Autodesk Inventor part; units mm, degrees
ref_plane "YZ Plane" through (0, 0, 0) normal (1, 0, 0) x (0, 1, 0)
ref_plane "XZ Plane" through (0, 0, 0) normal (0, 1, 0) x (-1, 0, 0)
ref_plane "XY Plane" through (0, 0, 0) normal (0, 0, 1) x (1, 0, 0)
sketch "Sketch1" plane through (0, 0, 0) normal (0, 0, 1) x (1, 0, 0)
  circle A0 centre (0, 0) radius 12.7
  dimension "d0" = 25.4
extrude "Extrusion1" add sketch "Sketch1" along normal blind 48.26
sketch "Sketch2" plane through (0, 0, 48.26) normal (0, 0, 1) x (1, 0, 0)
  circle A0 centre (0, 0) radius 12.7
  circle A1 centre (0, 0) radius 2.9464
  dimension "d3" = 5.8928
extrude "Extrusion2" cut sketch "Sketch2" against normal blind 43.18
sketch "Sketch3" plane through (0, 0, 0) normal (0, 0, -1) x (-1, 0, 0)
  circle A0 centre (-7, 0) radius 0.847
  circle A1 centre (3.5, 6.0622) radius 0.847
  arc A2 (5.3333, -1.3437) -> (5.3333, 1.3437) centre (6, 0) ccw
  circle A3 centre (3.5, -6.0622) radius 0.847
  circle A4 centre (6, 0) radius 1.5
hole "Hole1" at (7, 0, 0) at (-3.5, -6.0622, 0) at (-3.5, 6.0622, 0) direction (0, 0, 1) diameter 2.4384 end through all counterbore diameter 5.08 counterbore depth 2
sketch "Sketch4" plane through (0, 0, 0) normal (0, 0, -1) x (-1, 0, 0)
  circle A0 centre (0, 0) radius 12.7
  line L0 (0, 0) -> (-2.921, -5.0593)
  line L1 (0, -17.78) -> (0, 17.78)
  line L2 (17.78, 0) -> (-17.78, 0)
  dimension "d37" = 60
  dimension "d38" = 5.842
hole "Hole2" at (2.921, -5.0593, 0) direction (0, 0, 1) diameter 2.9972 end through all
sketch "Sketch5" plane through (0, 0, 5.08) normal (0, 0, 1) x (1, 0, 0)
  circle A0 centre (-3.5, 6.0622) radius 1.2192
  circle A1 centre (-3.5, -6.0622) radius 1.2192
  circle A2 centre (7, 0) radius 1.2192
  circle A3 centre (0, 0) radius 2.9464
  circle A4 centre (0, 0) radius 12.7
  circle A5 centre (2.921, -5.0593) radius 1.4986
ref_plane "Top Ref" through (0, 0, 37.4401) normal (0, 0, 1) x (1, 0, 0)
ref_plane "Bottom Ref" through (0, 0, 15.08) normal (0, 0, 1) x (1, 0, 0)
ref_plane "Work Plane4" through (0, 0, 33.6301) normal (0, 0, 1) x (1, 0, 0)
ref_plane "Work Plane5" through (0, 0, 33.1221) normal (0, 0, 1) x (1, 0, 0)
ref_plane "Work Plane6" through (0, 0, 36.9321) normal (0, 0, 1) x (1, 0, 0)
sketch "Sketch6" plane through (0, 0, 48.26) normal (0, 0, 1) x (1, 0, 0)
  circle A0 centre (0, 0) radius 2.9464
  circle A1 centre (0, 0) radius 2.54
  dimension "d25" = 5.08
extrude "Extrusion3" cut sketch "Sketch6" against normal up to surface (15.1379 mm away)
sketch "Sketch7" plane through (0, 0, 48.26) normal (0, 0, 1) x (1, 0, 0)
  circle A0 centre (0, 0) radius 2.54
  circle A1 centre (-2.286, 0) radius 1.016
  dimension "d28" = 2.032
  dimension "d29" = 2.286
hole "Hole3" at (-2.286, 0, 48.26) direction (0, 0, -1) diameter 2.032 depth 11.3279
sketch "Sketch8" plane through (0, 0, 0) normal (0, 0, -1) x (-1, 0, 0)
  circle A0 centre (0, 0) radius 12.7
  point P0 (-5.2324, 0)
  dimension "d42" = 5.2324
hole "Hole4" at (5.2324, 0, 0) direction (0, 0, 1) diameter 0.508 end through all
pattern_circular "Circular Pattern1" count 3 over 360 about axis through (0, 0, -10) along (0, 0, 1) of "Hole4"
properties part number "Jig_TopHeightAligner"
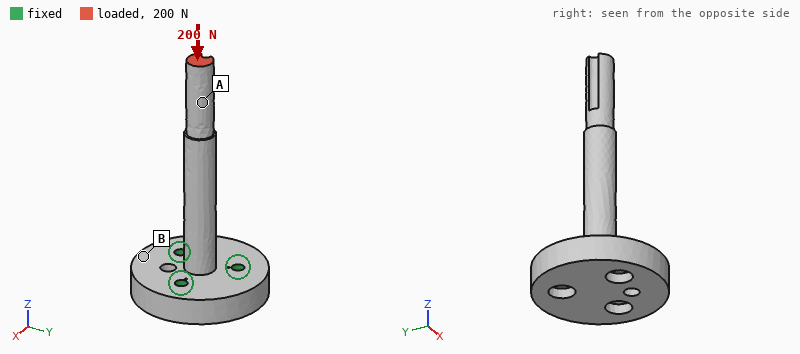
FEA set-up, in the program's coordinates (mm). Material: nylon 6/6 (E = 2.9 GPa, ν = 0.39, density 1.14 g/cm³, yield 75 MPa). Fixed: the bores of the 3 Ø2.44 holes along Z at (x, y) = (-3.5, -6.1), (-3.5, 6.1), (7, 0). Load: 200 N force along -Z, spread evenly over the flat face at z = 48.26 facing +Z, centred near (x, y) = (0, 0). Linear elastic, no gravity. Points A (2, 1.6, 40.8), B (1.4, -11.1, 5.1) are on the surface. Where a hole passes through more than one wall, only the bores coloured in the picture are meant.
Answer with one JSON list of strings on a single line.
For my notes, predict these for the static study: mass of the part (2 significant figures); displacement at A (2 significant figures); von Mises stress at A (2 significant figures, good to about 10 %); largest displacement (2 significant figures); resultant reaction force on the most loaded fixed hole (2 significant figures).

["3.9 g", "0.22 mm", "11 MPa", "0.30 mm", "71 N"]
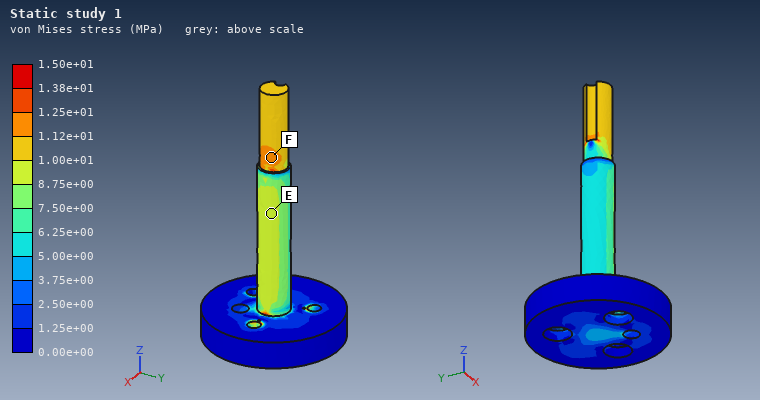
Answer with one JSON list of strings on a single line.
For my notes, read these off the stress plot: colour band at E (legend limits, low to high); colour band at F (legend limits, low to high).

["8.75e+00 to 1.00e+01 MPa", "1.12e+01 to 1.25e+01 MPa"]
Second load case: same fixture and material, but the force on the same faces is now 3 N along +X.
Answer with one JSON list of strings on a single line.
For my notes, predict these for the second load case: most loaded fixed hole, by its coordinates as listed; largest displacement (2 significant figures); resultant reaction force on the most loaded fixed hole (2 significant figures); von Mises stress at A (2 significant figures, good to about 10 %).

["(7, 0)", "0.55 mm", "12 N", "1.7 MPa"]
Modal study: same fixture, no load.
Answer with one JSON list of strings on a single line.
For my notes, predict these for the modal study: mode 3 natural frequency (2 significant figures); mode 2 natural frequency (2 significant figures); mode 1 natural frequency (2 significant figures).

["3900 Hz", "760 Hz", "760 Hz"]
